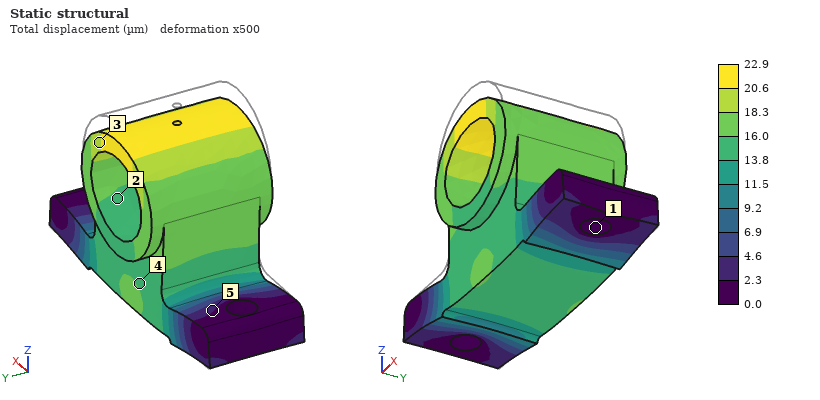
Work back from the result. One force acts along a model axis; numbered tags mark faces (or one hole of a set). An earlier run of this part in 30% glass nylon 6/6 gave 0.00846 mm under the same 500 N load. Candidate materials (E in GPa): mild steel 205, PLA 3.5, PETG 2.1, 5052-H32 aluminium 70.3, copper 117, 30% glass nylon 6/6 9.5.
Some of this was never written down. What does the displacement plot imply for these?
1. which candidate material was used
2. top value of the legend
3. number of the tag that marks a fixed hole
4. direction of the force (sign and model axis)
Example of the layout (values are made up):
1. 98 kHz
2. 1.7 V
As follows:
1. PLA
2. 22.9 µm
3. 1
4. -Z
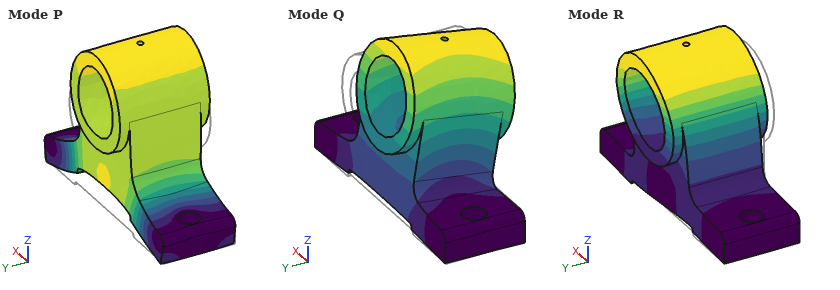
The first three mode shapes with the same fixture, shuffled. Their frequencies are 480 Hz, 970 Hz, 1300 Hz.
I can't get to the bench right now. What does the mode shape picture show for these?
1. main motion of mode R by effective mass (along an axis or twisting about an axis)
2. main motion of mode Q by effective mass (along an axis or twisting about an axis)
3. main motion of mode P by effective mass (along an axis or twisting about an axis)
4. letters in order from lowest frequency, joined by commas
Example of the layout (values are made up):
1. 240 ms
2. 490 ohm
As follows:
1. along X
2. along Y
3. along Z
4. Q, R, P
